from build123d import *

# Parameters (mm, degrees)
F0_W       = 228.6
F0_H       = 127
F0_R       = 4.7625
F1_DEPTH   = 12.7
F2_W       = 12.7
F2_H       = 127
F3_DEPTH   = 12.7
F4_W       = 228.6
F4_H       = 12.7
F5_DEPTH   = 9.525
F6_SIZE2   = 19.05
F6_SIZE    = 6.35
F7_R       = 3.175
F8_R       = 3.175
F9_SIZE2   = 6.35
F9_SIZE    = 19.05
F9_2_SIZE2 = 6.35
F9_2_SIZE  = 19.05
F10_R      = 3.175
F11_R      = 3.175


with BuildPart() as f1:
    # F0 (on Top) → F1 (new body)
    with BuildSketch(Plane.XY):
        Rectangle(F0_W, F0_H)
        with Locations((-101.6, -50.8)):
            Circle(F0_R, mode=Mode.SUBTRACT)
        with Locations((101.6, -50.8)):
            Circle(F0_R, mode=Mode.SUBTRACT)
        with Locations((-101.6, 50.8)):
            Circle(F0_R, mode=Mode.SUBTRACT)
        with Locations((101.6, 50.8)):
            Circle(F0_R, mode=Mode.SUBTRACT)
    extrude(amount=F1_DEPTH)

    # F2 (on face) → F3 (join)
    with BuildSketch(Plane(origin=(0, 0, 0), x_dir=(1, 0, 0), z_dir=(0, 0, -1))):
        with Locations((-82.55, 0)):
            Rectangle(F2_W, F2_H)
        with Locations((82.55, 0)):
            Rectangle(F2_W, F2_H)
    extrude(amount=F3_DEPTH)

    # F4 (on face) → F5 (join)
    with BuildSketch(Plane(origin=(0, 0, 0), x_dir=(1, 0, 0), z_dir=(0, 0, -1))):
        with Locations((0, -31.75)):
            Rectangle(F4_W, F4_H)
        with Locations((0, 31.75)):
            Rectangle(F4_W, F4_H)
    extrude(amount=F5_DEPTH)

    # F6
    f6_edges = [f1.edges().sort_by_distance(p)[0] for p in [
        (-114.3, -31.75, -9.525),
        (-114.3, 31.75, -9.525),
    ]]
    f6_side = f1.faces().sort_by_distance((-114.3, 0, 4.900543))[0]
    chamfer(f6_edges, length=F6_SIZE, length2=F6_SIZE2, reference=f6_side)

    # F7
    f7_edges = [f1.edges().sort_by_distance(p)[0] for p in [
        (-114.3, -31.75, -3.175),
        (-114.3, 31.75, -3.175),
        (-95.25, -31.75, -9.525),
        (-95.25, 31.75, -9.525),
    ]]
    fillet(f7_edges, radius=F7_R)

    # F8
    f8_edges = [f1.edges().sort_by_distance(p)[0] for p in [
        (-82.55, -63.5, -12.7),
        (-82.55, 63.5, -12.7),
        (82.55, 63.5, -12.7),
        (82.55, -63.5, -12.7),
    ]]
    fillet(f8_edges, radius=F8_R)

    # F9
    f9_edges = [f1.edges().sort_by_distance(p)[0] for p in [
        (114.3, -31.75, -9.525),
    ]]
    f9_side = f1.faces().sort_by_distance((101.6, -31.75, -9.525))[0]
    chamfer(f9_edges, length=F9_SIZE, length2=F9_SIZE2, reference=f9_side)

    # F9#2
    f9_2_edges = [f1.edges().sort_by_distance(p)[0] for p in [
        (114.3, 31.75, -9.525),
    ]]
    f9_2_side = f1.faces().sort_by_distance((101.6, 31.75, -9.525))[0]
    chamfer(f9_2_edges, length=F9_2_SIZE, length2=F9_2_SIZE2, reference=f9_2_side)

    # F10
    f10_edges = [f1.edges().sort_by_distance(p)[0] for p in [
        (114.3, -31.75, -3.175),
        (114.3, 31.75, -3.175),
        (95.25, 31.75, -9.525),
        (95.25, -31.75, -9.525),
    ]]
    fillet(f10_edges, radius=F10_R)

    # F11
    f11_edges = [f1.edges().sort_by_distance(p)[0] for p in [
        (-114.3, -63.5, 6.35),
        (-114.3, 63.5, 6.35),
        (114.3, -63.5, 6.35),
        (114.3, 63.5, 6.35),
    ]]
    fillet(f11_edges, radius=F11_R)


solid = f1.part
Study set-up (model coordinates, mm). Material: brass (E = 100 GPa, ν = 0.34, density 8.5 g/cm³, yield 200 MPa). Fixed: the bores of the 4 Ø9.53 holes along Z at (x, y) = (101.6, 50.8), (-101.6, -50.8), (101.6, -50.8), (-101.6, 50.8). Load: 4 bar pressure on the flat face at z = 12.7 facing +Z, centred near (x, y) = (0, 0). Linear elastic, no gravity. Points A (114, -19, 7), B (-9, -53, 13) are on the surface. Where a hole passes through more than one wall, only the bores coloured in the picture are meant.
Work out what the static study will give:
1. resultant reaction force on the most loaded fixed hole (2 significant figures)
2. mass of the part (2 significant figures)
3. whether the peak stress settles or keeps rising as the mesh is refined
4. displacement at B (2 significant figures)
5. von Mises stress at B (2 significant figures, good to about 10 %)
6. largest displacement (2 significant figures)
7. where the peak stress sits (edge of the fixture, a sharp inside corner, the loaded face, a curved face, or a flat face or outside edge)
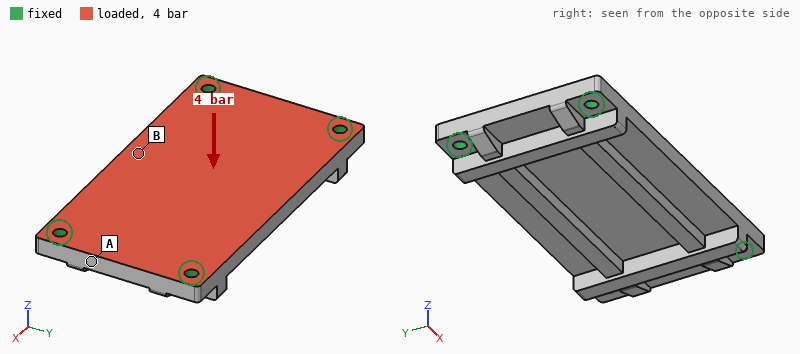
3.1 kN
3.8 kg
keeps rising
87 µm
19 MPa
91 µm
edge of the fixture
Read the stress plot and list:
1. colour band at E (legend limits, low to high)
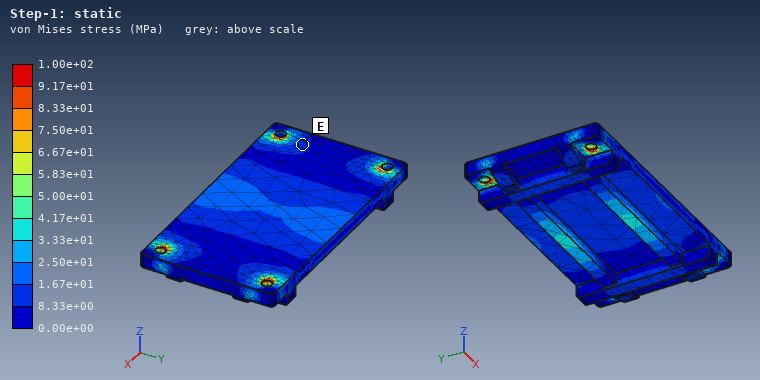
8.33e+00 to 1.67e+01 MPa
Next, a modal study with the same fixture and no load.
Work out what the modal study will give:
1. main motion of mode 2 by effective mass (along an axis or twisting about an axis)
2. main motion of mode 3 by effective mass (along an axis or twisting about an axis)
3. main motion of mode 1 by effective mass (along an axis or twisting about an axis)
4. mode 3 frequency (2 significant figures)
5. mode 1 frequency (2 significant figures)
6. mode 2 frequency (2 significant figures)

twisting about X
twisting about Y
along Z
2900 Hz
1100 Hz
1700 Hz
